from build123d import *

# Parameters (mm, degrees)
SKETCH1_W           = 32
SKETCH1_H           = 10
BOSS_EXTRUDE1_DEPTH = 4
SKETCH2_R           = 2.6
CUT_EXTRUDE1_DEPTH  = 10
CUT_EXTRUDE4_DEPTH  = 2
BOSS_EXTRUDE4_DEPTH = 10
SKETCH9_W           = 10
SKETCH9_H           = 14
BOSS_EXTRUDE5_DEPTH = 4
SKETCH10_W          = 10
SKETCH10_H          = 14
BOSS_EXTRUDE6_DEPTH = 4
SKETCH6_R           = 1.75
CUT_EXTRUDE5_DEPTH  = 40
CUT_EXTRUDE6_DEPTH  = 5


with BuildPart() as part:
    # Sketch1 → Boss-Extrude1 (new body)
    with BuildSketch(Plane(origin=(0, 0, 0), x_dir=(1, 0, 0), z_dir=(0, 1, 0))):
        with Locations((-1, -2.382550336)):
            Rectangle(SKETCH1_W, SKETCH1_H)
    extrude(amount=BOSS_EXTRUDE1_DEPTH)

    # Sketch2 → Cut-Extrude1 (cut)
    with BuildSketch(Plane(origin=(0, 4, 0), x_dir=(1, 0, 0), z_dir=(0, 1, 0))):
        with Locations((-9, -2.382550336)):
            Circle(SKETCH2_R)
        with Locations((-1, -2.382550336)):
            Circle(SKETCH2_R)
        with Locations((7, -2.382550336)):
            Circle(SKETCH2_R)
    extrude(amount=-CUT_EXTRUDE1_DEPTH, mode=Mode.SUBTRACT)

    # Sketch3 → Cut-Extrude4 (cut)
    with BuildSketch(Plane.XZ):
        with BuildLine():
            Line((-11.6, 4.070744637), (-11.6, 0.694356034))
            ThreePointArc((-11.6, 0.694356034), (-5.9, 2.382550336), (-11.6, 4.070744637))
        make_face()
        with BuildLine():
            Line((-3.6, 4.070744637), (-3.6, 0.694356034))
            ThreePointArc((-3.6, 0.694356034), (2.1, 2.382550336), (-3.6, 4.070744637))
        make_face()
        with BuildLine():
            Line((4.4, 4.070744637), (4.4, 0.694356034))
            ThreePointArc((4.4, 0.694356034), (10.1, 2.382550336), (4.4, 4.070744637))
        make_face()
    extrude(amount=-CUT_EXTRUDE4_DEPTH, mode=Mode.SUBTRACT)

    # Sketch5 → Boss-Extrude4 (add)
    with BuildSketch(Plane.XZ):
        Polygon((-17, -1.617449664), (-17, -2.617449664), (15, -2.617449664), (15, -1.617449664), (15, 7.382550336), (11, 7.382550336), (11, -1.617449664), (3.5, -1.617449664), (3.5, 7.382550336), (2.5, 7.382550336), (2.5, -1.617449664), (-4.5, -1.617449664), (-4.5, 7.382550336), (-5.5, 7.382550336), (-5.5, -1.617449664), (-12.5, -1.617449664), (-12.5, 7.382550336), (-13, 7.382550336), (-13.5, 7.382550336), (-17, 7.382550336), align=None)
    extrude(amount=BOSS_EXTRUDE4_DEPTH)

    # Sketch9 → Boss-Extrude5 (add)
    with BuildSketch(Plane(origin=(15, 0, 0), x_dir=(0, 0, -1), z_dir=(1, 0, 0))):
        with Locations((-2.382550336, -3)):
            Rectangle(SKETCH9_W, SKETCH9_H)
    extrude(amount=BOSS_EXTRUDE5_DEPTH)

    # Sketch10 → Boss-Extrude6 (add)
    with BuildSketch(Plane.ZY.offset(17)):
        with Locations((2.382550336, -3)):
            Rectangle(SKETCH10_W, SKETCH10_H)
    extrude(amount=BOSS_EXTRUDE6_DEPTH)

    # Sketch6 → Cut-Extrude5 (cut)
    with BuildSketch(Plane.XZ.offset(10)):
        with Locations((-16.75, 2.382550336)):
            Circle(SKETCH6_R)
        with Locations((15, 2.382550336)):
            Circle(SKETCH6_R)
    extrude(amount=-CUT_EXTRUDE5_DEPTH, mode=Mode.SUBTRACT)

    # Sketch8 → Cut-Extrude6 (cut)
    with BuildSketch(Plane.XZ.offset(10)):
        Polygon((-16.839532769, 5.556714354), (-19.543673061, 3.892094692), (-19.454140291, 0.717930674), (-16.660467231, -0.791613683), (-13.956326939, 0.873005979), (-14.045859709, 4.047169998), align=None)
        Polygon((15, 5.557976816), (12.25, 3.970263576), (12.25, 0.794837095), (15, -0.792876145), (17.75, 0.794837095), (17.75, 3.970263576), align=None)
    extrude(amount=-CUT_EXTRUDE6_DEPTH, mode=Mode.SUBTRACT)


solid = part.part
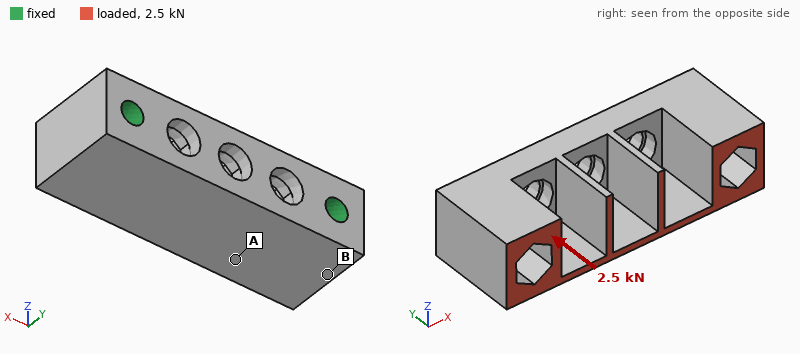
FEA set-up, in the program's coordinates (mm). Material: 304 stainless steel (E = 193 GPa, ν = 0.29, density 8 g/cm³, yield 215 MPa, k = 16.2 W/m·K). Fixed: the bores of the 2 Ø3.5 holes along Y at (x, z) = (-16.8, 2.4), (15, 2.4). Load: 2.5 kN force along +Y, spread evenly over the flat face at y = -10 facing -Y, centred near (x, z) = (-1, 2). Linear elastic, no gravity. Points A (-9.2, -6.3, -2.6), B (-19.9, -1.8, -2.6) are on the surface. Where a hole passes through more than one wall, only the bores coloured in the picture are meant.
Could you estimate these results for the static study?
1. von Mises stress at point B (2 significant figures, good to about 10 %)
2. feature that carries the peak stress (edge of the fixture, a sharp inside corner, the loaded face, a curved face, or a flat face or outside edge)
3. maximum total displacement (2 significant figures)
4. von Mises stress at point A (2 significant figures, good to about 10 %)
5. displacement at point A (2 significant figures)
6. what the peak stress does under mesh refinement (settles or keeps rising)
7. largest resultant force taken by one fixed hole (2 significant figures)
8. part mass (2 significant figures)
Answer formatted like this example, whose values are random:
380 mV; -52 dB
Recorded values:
9.1 MPa; edge of the fixture; 5.3 µm; 23 MPa; 2.3 µm; keeps rising; 1.3 kN; 23 g
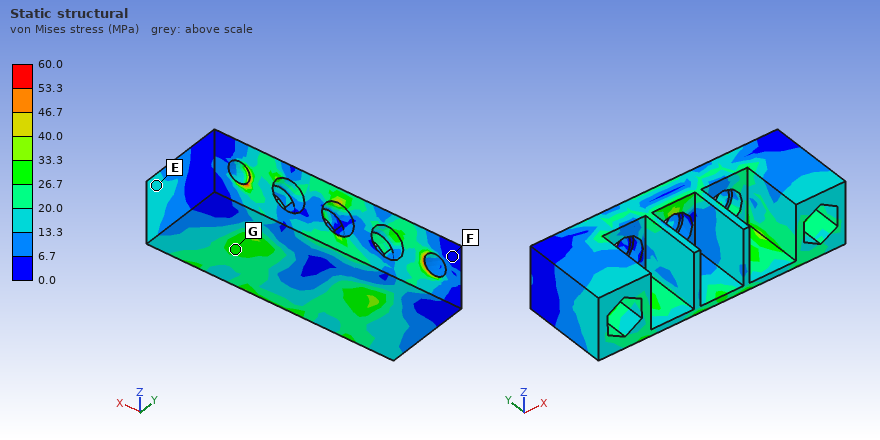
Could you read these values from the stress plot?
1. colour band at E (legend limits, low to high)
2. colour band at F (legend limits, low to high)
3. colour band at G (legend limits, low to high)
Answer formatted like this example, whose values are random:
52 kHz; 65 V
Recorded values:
13.3 to 20.0 MPa; 0.0 to 6.7 MPa; 26.7 to 33.3 MPa
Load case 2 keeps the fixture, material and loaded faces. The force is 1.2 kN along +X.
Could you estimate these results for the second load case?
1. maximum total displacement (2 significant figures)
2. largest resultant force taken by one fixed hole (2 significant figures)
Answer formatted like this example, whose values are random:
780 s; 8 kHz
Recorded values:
52 µm; 640 N
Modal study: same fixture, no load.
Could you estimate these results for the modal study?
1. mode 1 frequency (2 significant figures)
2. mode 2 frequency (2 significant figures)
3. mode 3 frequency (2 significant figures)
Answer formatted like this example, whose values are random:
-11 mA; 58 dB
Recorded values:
15 kHz; 16 kHz; 16 kHz
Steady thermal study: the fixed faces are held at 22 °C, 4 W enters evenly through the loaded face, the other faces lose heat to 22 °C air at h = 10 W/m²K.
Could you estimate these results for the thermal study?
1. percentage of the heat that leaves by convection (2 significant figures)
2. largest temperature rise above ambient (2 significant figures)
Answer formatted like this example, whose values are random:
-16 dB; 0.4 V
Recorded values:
5.1 %; 22 K
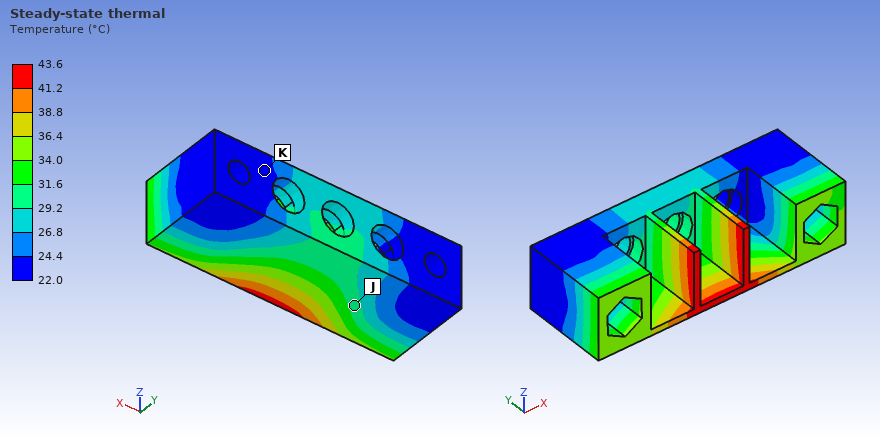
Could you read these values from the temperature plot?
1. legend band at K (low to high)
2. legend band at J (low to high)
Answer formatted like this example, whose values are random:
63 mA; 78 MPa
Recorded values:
22.0 to 24.4 °C; 29.2 to 31.6 °C
